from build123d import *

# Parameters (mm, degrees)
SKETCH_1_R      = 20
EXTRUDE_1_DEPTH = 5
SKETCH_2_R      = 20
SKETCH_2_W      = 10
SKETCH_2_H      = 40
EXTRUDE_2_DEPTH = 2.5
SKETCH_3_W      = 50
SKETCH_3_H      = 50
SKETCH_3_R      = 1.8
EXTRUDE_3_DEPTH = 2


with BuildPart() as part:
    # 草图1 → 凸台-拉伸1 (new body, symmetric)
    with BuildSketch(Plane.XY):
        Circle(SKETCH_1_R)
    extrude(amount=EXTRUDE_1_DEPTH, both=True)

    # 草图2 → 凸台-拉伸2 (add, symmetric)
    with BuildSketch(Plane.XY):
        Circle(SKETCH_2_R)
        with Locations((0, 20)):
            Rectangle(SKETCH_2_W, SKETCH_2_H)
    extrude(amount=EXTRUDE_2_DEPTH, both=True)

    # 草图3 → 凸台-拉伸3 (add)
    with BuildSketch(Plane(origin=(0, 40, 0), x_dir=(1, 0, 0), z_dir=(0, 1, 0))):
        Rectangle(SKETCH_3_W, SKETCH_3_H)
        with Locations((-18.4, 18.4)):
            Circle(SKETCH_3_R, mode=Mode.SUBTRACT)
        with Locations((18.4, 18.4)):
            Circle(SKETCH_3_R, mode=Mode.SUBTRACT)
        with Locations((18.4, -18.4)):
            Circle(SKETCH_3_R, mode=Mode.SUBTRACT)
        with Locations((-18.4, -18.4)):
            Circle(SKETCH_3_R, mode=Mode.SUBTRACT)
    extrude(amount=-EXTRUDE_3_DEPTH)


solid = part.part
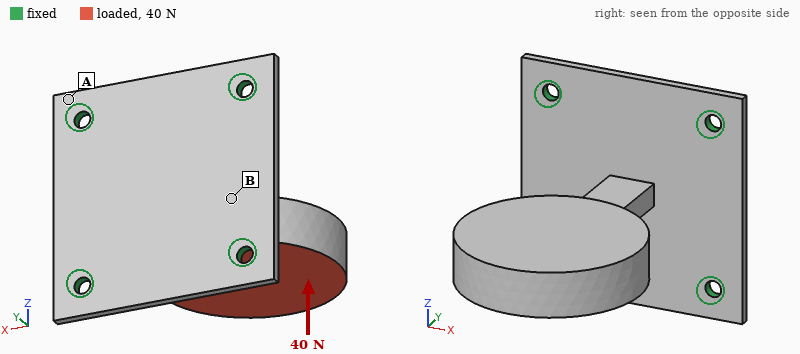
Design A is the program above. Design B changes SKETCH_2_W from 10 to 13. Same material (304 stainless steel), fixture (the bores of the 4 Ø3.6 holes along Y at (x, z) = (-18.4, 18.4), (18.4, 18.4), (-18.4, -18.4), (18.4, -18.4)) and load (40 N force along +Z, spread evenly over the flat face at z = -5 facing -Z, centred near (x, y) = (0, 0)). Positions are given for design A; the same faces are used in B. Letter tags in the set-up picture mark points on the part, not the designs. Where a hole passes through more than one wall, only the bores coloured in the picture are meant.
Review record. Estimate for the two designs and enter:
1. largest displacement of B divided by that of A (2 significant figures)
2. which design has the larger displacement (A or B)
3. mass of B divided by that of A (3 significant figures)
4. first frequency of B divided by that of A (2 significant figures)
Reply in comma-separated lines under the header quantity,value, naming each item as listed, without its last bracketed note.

quantity,value
largest displacement of B divided by that of A,0.84
which design has the larger displacement,A
mass of B divided by that of A,1.02
first frequency of B divided by that of A,1.1
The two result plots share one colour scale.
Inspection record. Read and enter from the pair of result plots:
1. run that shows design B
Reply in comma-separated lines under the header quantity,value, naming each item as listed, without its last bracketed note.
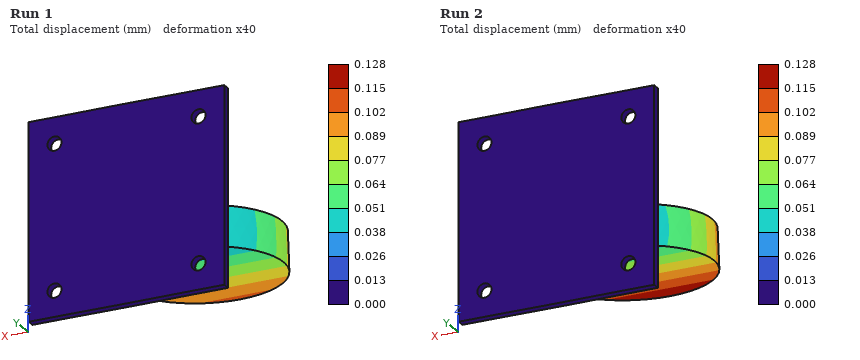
quantity,value
run that shows design B,Run 1
